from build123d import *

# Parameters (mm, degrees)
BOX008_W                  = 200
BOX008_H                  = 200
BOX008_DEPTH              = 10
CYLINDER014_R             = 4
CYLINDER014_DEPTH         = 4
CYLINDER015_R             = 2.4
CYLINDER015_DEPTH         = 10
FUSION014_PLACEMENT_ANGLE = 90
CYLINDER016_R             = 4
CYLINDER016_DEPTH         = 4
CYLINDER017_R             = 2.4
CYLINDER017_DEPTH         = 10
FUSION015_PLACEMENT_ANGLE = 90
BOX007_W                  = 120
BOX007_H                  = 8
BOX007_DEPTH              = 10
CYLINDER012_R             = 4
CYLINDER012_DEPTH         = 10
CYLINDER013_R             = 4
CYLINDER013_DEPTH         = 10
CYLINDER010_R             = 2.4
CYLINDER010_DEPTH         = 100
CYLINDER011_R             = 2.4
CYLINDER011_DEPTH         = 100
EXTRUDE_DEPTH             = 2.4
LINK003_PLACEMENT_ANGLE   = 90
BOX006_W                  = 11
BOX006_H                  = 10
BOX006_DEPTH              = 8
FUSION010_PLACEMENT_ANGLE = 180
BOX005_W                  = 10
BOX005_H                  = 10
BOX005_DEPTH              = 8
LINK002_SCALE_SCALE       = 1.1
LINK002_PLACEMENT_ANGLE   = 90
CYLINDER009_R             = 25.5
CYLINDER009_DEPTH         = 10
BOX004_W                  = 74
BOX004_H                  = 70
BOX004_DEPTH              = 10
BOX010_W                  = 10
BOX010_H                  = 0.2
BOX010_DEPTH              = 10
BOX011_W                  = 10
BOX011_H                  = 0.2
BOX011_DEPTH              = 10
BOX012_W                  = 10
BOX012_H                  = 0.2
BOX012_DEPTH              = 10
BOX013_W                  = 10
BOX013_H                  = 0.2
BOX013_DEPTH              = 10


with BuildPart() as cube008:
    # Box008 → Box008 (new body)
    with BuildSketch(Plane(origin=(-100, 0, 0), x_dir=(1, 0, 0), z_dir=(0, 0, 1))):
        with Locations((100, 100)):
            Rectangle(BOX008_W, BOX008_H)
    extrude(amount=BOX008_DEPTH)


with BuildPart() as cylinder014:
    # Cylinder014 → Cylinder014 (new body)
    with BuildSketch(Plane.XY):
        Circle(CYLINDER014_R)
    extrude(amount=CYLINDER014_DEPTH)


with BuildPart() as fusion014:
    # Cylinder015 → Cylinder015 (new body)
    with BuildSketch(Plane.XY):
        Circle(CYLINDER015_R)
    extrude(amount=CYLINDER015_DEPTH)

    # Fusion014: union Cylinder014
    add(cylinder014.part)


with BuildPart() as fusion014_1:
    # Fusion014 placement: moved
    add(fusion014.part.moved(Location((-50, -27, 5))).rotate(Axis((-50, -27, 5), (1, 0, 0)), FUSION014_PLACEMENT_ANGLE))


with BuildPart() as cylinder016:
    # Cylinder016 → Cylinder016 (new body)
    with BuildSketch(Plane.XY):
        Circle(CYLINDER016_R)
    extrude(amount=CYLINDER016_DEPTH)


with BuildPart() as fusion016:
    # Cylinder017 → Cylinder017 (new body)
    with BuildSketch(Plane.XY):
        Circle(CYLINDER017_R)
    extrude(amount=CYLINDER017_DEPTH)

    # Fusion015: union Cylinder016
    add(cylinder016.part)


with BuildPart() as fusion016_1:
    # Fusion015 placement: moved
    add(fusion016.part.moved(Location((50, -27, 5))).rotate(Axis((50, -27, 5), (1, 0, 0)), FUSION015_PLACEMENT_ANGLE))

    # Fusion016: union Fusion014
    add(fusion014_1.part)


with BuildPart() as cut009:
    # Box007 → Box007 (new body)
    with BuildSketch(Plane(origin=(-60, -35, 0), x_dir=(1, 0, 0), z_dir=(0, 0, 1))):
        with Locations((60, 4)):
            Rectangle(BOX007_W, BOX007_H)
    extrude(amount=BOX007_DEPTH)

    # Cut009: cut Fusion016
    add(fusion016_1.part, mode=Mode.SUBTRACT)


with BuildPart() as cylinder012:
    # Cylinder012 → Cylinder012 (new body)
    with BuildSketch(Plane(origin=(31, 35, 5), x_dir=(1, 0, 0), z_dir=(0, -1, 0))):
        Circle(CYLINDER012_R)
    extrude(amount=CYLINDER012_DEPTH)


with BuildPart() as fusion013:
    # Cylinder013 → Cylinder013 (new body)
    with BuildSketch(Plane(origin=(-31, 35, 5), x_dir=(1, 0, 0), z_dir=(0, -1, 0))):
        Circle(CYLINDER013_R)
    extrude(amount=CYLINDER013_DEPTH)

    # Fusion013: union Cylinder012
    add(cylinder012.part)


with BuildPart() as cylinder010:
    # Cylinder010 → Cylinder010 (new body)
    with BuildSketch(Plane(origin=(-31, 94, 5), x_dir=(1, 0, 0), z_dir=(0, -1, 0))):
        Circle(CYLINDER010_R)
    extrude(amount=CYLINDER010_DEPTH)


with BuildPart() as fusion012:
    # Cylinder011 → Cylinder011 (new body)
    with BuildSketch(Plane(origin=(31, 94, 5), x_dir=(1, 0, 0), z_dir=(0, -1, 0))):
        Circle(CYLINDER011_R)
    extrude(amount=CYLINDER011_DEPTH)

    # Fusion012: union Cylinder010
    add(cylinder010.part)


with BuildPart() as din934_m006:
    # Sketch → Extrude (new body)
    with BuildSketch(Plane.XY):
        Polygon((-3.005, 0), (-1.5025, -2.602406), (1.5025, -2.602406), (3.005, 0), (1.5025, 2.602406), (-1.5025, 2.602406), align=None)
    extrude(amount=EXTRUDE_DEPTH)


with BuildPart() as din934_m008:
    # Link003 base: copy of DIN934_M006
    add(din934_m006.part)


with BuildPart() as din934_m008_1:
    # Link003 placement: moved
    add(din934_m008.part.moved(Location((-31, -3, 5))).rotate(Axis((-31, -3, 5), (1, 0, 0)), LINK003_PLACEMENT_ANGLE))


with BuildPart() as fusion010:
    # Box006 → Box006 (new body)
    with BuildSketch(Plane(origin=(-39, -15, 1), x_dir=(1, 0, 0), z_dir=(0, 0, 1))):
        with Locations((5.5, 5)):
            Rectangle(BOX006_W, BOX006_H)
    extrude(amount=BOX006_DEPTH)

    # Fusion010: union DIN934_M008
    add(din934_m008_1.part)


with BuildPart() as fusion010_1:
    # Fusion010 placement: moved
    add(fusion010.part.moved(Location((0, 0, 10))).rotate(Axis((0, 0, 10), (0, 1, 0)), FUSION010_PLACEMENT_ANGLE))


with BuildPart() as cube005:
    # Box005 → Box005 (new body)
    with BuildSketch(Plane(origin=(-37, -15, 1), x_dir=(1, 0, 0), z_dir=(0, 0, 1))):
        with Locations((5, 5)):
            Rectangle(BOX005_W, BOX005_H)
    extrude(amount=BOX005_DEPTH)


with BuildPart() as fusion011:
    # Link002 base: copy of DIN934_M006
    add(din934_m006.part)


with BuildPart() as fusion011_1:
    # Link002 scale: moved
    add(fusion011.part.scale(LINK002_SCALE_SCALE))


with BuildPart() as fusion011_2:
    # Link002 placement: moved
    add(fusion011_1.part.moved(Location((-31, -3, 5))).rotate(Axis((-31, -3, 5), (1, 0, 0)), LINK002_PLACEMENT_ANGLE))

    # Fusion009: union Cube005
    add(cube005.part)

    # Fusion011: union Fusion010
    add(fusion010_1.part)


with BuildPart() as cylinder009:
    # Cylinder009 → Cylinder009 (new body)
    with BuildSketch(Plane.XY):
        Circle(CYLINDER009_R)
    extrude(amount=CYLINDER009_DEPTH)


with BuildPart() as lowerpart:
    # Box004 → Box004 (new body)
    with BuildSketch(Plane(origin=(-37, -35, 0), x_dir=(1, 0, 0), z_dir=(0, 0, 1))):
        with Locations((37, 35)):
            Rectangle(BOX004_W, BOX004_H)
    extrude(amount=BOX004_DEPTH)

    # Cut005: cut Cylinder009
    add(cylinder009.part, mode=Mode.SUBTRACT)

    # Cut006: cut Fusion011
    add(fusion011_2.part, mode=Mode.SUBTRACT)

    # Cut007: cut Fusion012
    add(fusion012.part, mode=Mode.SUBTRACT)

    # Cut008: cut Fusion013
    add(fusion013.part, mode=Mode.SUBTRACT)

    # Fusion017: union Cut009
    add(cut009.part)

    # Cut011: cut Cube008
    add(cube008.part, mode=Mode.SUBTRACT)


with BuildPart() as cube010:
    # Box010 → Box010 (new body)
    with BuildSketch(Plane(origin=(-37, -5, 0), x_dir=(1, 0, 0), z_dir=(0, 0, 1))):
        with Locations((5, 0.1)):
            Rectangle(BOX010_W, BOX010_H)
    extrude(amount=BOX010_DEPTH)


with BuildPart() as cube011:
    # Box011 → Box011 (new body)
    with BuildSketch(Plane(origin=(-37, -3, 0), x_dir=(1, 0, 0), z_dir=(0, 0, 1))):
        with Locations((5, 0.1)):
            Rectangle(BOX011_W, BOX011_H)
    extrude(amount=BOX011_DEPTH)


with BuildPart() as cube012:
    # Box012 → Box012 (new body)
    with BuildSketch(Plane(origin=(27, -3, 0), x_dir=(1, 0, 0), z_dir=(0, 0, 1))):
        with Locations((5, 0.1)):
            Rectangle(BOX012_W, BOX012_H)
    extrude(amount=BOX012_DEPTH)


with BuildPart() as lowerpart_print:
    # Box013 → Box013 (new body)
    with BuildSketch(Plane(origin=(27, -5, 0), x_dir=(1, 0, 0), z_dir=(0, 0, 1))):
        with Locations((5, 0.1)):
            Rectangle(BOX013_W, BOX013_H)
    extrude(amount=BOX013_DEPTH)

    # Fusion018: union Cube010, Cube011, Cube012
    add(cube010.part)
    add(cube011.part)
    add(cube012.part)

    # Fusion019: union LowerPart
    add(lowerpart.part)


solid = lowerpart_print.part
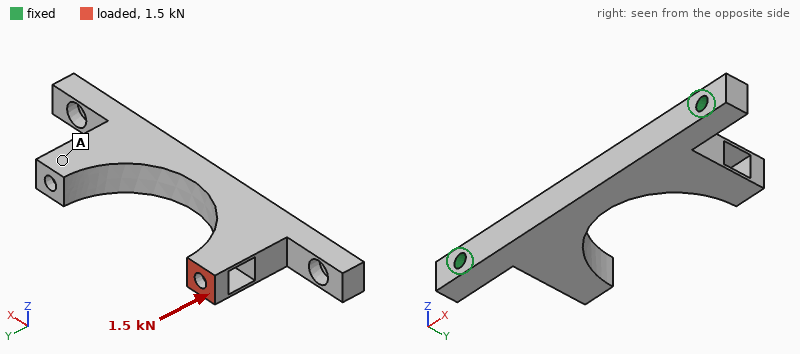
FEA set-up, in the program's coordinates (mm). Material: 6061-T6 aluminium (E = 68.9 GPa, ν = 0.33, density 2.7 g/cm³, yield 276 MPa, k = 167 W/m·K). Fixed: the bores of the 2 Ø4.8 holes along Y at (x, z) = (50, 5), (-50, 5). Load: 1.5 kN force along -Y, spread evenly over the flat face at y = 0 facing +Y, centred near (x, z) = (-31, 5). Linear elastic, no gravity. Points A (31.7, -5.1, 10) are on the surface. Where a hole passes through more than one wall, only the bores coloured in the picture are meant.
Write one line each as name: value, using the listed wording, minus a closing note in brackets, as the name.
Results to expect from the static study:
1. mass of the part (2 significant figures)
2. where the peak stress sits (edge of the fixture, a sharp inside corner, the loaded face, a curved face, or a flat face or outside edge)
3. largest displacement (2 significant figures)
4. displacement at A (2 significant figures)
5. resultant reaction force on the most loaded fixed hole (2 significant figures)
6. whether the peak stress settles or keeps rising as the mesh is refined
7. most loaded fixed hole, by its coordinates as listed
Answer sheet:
mass of the part: 46 g
where the peak stress sits: edge of the fixture
largest displacement: 75 µm
displacement at A: 46 µm
resultant reaction force on the most loaded fixed hole: 1.5 kN
whether the peak stress settles or keeps rising as the mesh is refined: keeps rising
most loaded fixed hole, by its coordinates as listed: (-50, 5)
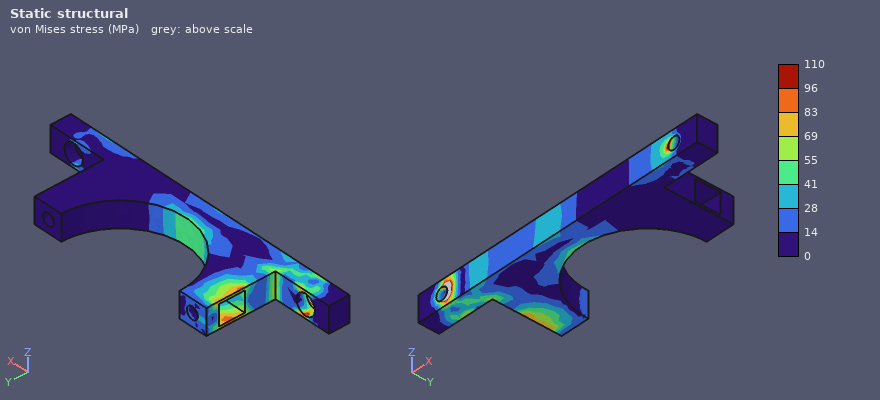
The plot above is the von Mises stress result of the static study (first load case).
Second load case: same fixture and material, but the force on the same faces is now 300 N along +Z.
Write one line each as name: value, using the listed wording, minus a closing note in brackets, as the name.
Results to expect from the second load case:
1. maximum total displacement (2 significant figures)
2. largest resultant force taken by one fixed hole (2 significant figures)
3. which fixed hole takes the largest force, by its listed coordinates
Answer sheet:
maximum total displacement: 0.24 mm
largest resultant force taken by one fixed hole: 270 N
which fixed hole takes the largest force, by its listed coordinates: (-50, 5)
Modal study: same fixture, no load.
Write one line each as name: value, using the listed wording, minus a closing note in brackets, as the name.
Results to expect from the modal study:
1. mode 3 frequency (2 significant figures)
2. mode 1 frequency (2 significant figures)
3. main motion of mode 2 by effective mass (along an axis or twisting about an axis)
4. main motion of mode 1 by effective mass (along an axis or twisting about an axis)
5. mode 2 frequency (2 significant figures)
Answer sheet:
mode 3 frequency: 4500 Hz
mode 1 frequency: 2600 Hz
main motion of mode 2 by effective mass: along Y
main motion of mode 1 by effective mass: along Z
mode 2 frequency: 3300 Hz
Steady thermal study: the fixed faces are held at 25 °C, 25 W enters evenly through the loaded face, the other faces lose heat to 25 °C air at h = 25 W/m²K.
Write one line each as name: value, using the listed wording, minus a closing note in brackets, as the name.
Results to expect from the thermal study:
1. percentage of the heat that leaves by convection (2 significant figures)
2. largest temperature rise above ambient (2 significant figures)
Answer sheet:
percentage of the heat that leaves by convection: 15 %
largest temperature rise above ambient: 75 K
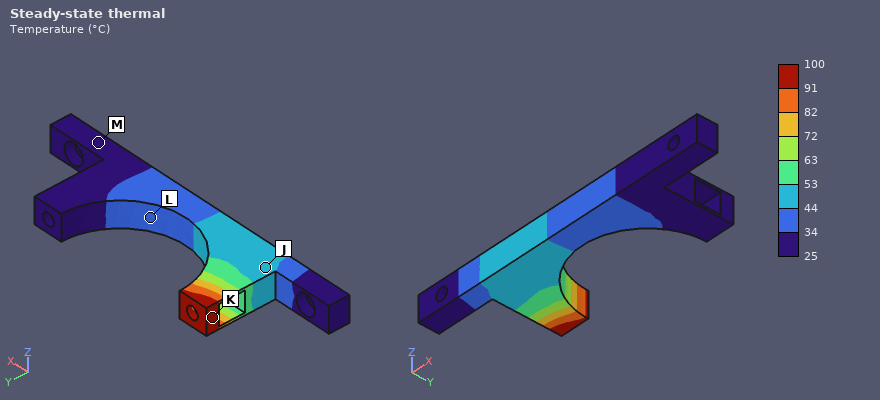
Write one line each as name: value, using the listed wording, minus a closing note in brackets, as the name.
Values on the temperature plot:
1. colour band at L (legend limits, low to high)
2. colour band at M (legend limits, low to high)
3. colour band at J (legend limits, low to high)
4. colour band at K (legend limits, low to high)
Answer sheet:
colour band at L: 34 to 44 °C
colour band at M: 25 to 34 °C
colour band at J: 44 to 53 °C
colour band at K: 91 to 100 °C
